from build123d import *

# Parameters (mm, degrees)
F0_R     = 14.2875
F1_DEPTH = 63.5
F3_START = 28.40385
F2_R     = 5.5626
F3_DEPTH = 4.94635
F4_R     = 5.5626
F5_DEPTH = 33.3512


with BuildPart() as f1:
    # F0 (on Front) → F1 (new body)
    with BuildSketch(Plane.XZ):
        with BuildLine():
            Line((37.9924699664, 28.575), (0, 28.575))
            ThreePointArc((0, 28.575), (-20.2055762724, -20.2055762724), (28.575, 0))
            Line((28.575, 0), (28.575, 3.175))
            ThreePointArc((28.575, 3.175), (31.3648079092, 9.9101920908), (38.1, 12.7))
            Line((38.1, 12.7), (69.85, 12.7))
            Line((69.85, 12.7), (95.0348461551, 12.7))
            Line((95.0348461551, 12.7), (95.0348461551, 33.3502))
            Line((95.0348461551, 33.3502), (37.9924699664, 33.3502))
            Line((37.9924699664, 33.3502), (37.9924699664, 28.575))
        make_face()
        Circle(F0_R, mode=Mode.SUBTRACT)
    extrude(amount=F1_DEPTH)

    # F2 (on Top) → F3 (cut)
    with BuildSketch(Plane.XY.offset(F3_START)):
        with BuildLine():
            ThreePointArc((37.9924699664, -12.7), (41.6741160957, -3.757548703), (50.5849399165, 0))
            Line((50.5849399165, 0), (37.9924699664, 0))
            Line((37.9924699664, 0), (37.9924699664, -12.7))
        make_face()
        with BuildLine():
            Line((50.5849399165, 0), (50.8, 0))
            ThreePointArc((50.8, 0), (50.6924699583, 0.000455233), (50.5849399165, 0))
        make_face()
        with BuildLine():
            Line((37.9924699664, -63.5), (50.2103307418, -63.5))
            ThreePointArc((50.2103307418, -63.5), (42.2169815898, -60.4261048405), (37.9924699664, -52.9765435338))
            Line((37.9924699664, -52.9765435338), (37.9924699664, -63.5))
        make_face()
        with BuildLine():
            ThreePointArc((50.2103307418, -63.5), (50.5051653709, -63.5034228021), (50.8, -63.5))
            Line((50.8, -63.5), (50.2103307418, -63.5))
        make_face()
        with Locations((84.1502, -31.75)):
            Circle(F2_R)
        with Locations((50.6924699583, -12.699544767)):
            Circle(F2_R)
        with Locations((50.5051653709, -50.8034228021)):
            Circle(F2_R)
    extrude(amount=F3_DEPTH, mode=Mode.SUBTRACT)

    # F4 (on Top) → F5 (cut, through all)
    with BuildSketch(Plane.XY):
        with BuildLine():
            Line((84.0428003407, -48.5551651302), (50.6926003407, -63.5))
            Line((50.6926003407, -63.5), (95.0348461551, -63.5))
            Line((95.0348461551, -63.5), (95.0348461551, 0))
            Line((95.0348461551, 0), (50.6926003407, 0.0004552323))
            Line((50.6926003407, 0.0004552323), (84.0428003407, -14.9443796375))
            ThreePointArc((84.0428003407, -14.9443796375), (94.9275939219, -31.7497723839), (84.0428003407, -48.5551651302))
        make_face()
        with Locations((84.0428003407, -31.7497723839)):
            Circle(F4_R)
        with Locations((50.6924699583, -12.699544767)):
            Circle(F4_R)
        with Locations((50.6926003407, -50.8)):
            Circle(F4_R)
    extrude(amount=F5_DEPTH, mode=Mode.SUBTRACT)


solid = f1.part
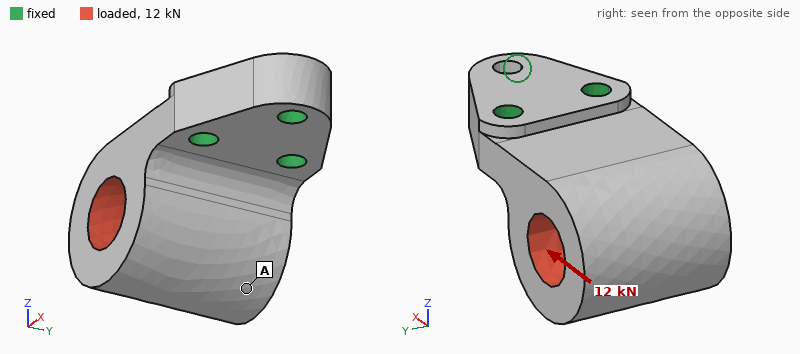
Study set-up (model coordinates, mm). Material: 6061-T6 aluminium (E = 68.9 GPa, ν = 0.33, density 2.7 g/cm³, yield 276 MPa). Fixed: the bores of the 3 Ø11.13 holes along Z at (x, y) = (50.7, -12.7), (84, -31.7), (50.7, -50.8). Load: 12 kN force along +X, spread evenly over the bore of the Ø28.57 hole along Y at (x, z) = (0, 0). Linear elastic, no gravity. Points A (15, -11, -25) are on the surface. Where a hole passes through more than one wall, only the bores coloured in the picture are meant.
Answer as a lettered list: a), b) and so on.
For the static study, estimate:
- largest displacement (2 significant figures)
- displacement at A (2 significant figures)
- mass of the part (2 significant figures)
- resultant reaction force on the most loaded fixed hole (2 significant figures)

a) 0.26 mm
b) 0.19 mm
c) 520 g
d) 5.9 kN
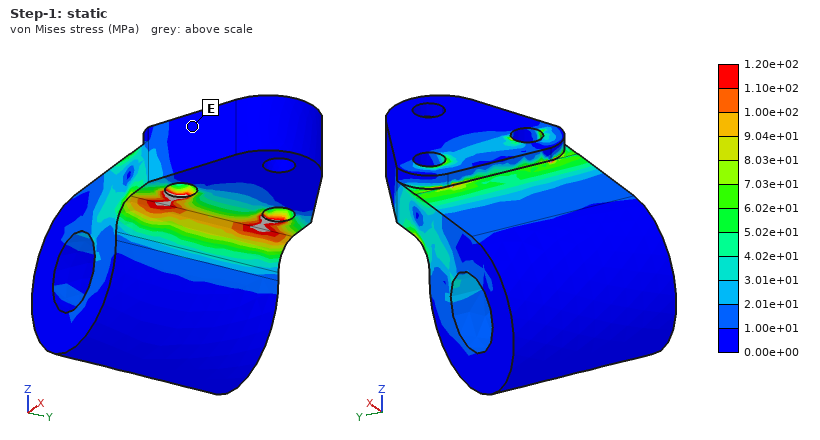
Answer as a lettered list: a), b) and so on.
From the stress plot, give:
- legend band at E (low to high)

a) 0.00e+00 to 1.00e+01 MPa
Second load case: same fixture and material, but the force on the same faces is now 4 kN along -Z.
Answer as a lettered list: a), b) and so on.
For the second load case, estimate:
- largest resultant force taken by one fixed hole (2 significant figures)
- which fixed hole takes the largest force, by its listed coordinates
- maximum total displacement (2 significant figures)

a) 2.5 kN
b) (50.7, -12.7)
c) 0.15 mm
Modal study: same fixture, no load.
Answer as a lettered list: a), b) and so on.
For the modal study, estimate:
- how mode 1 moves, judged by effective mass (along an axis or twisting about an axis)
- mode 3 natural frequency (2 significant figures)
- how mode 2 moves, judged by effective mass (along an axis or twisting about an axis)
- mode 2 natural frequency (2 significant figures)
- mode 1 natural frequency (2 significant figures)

a) along Z
b) 5500 Hz
c) along Y
d) 3600 Hz
e) 1500 Hz
